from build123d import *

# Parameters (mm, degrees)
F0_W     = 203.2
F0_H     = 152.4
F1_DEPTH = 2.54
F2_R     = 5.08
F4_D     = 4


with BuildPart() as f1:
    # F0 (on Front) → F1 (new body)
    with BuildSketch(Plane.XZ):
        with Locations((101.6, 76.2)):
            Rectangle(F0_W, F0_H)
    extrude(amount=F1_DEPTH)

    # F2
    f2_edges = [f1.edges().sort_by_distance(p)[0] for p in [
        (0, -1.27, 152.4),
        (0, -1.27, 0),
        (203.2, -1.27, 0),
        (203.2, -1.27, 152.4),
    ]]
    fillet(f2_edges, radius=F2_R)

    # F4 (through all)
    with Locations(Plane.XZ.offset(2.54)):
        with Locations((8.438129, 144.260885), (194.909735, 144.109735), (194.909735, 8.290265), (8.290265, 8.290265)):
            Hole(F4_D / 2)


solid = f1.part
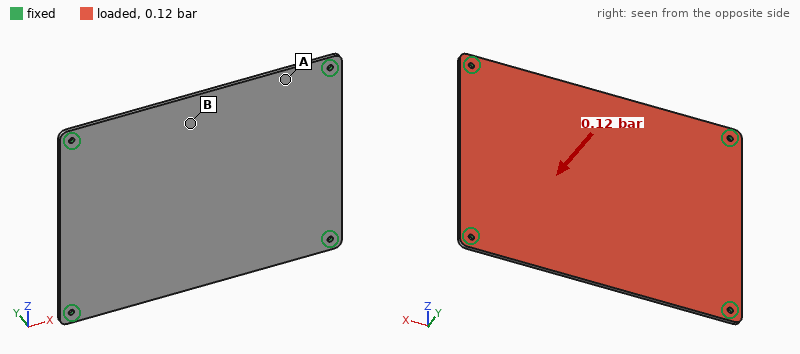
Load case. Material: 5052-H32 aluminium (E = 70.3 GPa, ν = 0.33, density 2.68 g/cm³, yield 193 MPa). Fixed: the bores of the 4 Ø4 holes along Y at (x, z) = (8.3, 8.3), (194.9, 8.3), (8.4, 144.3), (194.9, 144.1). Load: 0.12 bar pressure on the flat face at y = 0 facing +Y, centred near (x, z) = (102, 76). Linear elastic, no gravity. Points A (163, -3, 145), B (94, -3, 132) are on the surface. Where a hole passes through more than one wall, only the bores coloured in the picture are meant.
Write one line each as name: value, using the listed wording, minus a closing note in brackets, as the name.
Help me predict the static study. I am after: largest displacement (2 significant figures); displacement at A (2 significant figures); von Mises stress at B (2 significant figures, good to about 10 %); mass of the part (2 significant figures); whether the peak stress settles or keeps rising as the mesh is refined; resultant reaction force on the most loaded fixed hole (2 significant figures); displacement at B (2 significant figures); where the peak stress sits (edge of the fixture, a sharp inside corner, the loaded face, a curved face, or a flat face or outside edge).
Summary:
largest displacement: 0.76 mm
displacement at A: 0.24 mm
von Mises stress at B: 21 MPa
mass of the part: 210 g
whether the peak stress settles or keeps rising as the mesh is refined: keeps rising
resultant reaction force on the most loaded fixed hole: 93 N
displacement at B: 0.67 mm
where the peak stress sits: edge of the fixture
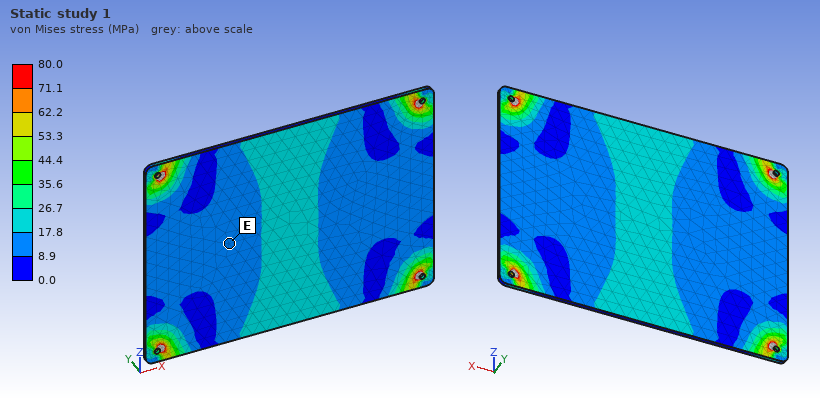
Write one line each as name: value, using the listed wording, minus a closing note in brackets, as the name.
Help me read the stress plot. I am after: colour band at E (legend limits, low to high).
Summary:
colour band at E: 8.9 to 17.8 MPa
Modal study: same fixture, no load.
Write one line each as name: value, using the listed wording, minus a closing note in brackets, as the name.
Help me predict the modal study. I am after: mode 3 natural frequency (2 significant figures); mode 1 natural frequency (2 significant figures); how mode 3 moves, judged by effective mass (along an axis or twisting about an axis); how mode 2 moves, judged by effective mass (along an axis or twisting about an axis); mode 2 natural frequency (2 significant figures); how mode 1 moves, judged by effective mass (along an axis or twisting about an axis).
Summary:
mode 3 natural frequency: 650 Hz
mode 1 natural frequency: 280 Hz
how mode 3 moves, judged by effective mass: twisting about Z
how mode 2 moves, judged by effective mass: twisting about X
mode 2 natural frequency: 480 Hz
how mode 1 moves, judged by effective mass: along Y
